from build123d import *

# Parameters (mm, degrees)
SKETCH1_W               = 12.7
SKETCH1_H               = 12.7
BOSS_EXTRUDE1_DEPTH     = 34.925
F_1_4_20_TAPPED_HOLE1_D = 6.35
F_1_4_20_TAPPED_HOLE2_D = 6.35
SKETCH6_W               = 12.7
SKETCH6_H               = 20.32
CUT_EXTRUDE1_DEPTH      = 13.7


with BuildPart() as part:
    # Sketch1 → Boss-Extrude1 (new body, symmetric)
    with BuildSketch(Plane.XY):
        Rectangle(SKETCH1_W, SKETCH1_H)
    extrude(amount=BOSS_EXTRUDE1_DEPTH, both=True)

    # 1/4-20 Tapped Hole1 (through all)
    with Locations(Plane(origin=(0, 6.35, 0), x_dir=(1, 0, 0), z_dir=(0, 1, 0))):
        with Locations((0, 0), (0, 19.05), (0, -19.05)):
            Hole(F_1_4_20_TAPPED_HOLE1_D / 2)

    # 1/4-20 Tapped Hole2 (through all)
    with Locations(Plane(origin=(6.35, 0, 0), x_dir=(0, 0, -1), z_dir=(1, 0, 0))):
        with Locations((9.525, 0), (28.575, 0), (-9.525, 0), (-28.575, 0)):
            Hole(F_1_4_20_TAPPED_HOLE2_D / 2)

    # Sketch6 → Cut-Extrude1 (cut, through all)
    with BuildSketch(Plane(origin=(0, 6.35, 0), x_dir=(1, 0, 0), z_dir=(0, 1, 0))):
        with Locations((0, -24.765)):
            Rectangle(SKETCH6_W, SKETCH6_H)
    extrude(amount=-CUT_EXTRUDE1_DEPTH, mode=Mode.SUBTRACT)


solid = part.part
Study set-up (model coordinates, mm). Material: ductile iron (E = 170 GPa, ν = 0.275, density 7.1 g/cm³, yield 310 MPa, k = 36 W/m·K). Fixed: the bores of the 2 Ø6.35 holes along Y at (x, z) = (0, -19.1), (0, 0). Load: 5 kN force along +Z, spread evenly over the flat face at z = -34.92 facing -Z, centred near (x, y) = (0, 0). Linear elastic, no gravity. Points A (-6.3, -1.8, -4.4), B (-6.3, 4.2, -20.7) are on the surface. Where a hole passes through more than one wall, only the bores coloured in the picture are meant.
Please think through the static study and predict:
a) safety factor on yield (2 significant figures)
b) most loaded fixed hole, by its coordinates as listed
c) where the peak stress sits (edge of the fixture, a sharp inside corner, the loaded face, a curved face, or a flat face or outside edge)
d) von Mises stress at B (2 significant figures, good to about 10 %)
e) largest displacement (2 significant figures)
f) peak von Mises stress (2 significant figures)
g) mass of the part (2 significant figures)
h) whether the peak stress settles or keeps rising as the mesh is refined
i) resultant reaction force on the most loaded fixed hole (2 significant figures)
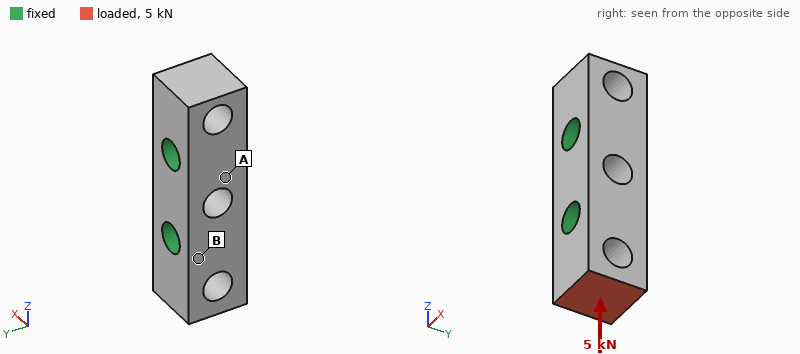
2.0
(0, -19.1)
a curved face
25 MPa
6.4 µm
150 MPa
42 g
settles
4.9 kN
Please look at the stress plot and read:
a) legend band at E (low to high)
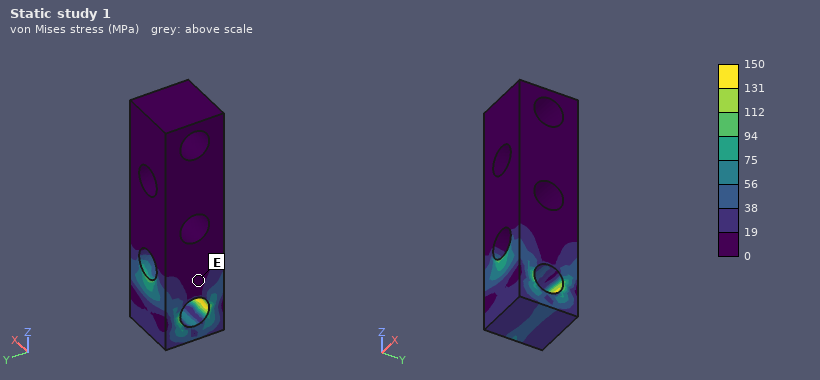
0 to 19 MPa
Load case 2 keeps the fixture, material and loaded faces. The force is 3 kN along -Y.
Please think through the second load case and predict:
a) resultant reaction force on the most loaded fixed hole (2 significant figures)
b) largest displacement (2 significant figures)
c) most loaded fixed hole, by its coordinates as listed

3.0 kN
24 µm
(0, -19.1)
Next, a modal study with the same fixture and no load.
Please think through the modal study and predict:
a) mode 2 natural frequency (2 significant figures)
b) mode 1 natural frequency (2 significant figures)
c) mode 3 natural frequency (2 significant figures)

28 kHz
28 kHz
32 kHz
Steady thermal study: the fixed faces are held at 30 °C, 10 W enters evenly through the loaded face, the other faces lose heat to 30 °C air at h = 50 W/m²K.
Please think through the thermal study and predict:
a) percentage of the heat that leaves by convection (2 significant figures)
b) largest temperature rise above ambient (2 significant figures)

7.4 %
34 K
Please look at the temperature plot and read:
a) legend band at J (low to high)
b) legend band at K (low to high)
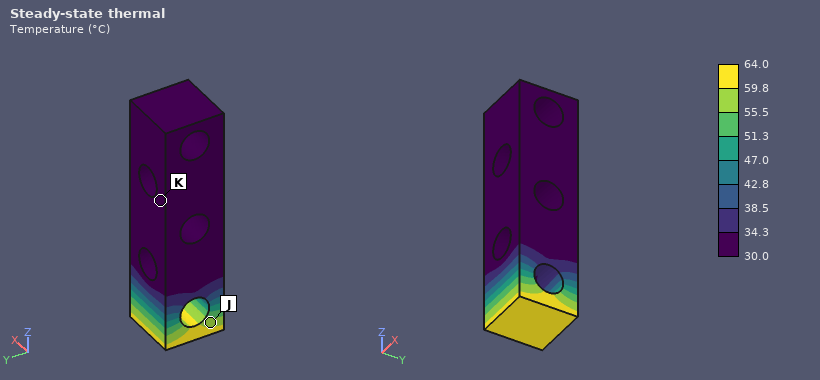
55.5 to 59.8 °C
30.0 to 34.3 °C
